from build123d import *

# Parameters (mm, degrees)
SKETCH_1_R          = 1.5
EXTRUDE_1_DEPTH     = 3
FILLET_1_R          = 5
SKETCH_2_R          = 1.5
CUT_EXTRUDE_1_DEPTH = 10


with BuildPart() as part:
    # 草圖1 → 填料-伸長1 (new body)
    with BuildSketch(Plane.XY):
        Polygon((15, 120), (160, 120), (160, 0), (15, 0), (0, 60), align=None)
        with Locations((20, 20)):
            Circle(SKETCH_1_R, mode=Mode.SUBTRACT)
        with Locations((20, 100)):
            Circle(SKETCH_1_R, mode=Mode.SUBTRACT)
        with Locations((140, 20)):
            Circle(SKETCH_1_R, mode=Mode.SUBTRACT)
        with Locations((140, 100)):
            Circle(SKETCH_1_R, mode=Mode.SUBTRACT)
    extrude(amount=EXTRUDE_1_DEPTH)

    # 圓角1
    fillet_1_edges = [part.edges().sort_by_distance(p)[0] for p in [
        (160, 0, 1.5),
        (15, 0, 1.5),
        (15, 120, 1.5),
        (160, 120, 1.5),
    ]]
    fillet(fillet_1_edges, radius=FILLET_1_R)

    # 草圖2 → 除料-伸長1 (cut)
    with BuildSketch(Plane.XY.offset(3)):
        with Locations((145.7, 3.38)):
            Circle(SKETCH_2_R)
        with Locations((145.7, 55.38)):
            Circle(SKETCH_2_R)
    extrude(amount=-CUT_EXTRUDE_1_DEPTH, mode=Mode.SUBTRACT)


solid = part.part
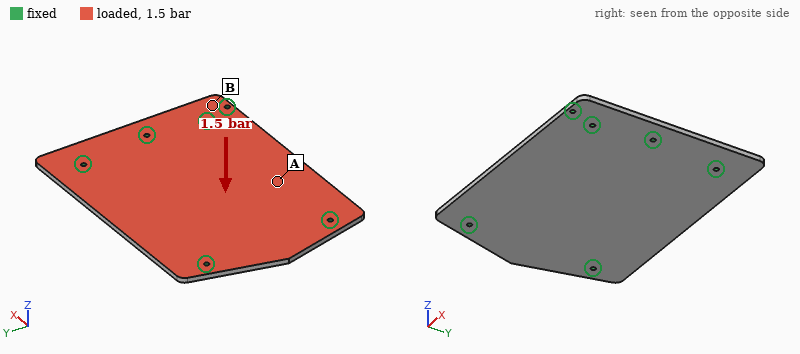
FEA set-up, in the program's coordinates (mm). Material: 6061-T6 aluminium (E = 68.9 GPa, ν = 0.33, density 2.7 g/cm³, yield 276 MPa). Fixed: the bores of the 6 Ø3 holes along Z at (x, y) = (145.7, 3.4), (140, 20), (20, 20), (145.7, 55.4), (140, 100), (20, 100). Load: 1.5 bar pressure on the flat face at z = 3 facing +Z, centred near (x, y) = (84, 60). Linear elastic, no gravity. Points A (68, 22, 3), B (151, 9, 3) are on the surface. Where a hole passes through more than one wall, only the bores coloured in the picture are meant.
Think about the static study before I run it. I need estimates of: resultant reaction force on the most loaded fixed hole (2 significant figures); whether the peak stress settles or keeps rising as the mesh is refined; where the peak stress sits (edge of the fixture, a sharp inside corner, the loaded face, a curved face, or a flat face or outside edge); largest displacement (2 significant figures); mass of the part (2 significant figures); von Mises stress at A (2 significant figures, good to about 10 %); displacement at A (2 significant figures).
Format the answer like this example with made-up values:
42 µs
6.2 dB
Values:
640 N
keeps rising
edge of the fixture
0.74 mm
150 g
63 MPa
0.66 mm
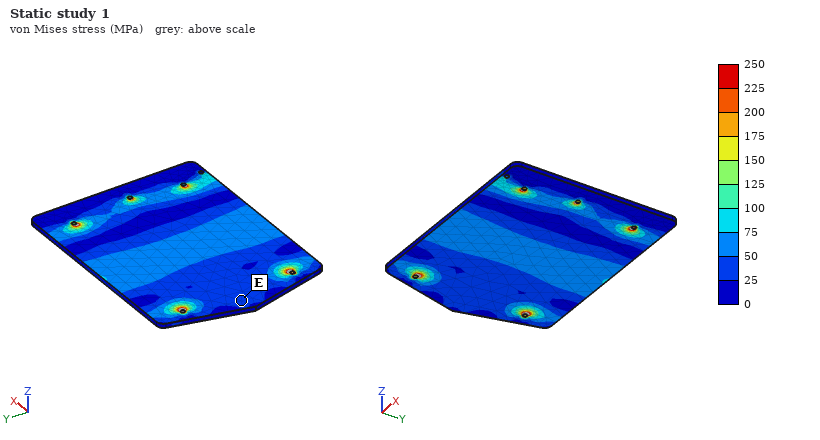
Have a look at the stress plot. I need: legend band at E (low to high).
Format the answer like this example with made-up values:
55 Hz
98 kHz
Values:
25 to 50 MPa
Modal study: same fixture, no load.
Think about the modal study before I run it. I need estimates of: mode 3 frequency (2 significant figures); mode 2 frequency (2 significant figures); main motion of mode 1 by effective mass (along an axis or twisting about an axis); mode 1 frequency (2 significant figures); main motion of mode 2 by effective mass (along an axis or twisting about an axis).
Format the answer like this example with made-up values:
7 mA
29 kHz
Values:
1800 Hz
1200 Hz
along Z
910 Hz
twisting about X
